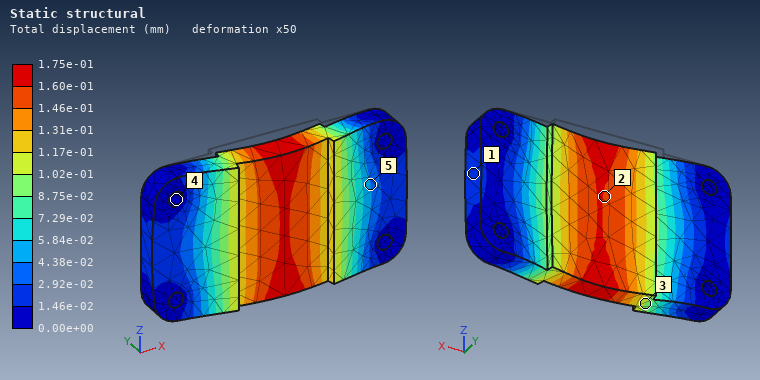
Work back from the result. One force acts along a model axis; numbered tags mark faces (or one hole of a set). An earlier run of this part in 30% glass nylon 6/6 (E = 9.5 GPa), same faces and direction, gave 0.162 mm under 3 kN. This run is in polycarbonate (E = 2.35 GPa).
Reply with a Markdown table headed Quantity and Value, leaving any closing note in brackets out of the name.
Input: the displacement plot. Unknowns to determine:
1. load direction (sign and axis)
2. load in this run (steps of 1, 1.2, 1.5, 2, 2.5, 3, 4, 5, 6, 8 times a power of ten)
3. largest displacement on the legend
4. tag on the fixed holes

| Quantity | Value |
|---|---|
| load direction | -Y |
| load in this run | 800 N |
| largest displacement on the legend | 1.75e-01 mm |
| tag on the fixed holes | 4 |
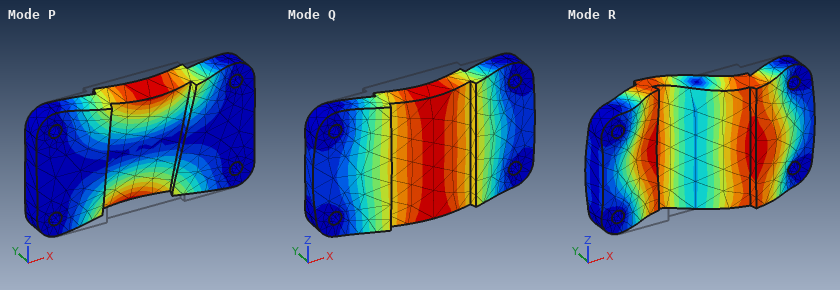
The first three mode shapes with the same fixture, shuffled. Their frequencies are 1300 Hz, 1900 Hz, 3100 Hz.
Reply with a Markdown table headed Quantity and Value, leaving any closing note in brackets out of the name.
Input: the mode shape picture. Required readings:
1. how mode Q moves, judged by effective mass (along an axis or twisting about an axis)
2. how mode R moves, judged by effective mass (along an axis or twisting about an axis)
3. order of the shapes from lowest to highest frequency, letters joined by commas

| Quantity | Value |
|---|---|
| how mode Q moves, judged by effective mass | along Y |
| how mode R moves, judged by effective mass | twisting about Z |
| order of the shapes from lowest to highest frequency, letters joined by commas | Q, P, R |
